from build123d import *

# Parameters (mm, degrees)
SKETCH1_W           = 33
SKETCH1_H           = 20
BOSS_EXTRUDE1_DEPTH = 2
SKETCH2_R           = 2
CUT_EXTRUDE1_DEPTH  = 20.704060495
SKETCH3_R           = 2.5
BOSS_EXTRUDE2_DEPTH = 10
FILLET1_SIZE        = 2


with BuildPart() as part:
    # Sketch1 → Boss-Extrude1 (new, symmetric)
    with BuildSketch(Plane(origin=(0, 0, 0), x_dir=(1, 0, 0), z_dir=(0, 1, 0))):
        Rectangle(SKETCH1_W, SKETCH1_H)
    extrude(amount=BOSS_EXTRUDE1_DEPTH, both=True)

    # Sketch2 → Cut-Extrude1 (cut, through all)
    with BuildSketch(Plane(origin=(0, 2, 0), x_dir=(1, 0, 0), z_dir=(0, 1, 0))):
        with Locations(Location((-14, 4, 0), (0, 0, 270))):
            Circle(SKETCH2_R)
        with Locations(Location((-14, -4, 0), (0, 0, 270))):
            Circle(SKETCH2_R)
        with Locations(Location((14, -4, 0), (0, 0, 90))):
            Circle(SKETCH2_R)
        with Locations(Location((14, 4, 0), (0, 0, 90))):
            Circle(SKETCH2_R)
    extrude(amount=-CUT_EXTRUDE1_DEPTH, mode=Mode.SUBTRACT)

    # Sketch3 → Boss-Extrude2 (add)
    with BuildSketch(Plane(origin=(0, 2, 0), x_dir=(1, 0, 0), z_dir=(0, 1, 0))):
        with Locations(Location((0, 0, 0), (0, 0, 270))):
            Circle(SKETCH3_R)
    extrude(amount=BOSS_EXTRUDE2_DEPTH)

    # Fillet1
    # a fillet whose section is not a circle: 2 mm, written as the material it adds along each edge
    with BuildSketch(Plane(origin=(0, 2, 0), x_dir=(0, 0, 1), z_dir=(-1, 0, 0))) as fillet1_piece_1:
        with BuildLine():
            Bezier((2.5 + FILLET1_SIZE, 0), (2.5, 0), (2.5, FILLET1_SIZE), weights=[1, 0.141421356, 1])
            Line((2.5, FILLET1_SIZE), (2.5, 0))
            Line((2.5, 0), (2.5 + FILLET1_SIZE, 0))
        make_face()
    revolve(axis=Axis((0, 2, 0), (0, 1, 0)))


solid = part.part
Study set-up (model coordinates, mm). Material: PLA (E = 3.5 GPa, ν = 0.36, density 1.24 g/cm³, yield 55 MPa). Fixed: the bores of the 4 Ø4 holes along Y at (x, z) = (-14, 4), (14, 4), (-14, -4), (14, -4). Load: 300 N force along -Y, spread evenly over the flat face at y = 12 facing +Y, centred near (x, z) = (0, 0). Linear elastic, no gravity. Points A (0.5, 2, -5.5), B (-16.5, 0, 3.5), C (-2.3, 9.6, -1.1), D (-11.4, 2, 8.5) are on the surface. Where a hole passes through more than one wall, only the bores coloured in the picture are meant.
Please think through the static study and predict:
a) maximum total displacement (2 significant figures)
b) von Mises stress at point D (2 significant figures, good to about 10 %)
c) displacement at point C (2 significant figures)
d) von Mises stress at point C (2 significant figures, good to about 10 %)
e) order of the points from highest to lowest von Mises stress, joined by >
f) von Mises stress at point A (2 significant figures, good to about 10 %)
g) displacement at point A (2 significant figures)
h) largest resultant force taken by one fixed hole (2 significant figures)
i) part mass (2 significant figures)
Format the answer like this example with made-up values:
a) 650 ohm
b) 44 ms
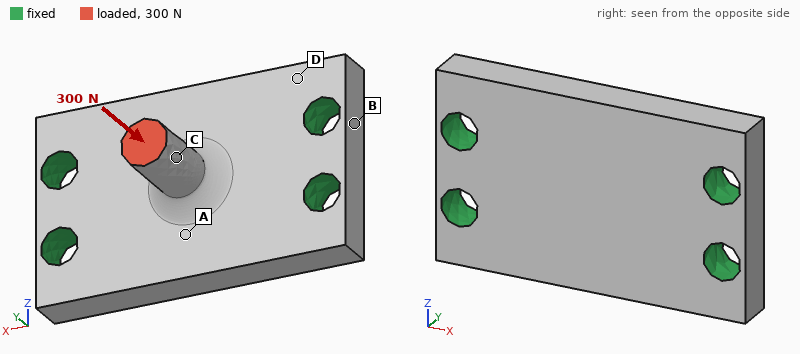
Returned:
a) 0.11 mm
b) 5.1 MPa
c) 0.10 mm
d) 15 MPa
e) C > A > D > B
f) 8.8 MPa
g) 0.068 mm
h) 76 N
i) 3.3 g
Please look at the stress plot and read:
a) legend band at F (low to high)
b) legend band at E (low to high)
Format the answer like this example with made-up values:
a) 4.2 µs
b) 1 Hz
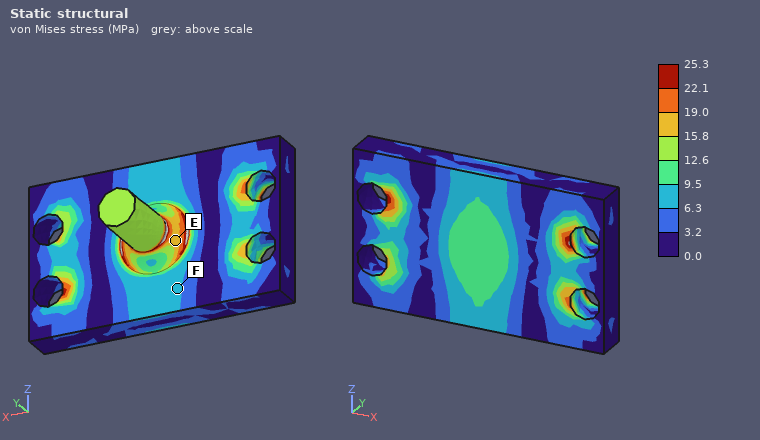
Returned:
a) 6.3 to 9.5 MPa
b) 15.8 to 19.0 MPa
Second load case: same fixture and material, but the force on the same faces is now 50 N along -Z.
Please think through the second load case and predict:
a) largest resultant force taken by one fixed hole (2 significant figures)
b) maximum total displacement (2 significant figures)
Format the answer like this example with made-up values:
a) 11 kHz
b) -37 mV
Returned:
a) 29 N
b) 0.21 mm
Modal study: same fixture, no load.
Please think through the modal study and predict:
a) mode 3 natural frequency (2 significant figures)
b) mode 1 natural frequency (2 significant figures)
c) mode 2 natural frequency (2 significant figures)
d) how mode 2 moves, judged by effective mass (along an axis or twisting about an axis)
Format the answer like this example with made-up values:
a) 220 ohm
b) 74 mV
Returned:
a) 10 kHz
b) 7900 Hz
c) 8500 Hz
d) along Y
